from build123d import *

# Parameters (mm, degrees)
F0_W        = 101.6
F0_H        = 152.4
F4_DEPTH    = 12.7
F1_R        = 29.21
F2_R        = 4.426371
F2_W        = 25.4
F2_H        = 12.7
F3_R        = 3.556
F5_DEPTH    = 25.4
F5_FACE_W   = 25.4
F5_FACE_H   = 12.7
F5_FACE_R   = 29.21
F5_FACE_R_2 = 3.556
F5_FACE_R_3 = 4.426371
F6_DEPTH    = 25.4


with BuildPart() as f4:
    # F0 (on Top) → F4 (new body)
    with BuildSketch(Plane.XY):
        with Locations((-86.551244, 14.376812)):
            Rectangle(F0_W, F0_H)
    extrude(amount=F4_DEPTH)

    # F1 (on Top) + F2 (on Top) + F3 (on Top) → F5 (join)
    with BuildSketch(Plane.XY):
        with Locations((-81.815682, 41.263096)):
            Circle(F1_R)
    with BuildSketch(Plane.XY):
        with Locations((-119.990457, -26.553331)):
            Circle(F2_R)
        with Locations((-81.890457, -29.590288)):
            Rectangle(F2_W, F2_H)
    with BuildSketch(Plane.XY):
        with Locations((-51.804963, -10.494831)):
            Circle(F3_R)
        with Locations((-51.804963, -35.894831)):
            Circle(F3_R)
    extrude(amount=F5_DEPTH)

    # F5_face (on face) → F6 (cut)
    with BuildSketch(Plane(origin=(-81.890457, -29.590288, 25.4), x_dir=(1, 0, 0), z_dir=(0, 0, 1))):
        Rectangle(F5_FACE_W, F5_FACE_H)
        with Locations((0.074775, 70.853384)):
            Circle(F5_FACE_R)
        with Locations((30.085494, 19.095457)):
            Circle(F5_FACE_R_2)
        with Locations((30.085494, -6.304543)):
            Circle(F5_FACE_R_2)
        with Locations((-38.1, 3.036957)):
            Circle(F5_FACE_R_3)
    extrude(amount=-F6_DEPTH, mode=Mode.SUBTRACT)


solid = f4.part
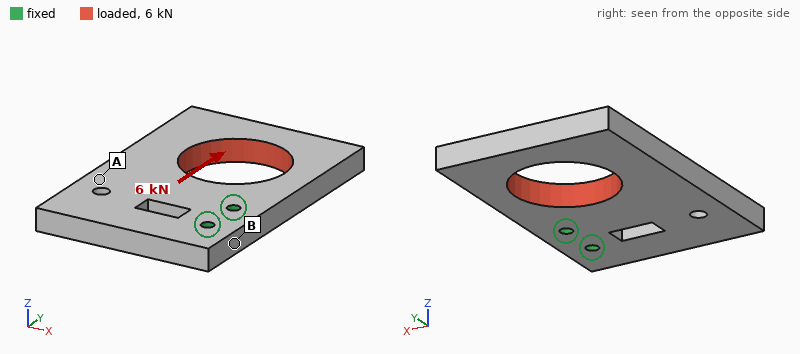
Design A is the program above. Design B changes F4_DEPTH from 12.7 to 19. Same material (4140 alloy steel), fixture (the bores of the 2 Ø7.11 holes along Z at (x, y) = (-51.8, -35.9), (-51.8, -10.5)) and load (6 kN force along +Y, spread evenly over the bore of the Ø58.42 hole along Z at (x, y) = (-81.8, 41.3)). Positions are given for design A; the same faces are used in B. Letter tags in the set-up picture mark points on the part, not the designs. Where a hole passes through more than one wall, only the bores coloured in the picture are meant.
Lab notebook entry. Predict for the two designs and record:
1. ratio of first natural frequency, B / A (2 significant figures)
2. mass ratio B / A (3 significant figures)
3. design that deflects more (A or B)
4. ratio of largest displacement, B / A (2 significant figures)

1.4
1.50
A
0.67
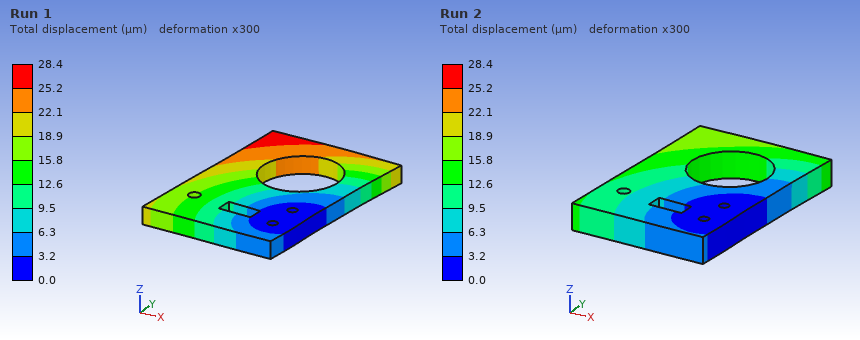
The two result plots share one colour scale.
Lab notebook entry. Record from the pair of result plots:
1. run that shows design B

Run 2
